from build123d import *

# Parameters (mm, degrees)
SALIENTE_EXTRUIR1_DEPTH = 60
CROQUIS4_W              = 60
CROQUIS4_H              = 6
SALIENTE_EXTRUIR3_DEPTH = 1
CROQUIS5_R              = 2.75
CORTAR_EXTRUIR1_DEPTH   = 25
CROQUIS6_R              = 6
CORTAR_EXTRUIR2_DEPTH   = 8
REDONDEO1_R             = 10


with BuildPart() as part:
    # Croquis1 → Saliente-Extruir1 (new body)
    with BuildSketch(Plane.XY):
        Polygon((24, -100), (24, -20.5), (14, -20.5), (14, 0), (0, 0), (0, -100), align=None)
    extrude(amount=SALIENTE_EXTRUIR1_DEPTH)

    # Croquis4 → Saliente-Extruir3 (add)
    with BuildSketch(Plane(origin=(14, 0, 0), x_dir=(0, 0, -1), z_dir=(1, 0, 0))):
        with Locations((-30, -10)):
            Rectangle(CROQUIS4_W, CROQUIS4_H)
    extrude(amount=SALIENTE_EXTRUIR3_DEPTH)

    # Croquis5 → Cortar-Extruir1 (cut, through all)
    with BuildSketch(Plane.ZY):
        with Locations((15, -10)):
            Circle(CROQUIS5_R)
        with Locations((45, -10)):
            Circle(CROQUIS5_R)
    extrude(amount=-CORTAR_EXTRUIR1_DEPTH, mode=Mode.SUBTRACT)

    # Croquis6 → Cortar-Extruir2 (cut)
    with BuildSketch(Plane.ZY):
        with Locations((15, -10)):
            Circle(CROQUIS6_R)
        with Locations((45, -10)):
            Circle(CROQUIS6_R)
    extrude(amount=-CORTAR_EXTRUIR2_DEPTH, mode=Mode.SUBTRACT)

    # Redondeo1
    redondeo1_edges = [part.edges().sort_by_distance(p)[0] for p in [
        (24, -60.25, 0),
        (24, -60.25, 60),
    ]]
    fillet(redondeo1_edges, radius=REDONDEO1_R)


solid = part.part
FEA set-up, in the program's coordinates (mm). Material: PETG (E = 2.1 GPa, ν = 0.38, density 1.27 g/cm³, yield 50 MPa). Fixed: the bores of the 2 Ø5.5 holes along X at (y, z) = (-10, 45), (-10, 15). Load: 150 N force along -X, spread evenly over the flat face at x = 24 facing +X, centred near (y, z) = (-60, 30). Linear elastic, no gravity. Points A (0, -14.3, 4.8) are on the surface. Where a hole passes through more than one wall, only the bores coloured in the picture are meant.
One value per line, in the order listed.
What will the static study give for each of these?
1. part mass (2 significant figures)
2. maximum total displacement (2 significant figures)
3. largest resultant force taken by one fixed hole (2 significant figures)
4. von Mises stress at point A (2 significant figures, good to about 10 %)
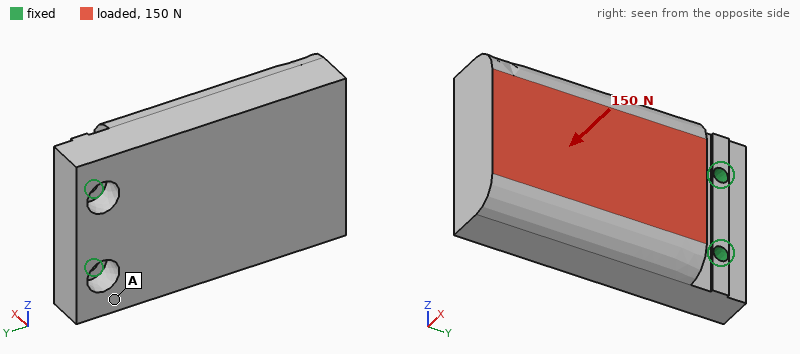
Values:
160 g
1.2 mm
80 N
3.7 MPa
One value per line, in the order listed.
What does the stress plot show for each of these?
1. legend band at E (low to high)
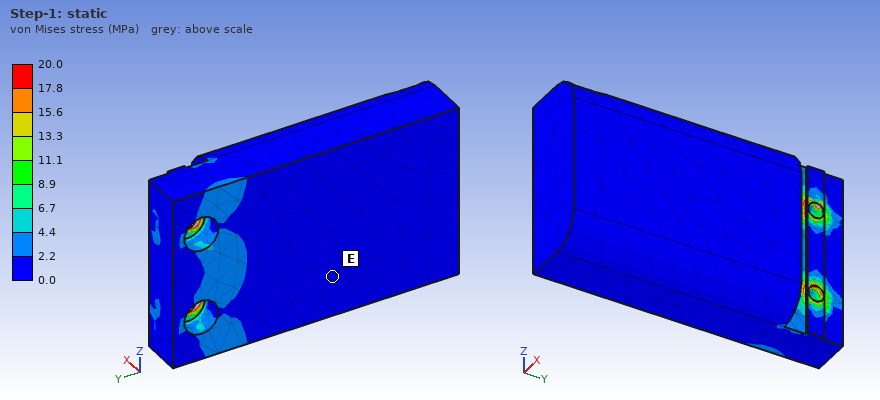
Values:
0.0 to 2.2 MPa
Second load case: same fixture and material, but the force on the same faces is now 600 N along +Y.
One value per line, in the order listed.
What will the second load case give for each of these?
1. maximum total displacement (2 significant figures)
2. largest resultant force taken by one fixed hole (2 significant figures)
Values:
1.4 mm
310 N
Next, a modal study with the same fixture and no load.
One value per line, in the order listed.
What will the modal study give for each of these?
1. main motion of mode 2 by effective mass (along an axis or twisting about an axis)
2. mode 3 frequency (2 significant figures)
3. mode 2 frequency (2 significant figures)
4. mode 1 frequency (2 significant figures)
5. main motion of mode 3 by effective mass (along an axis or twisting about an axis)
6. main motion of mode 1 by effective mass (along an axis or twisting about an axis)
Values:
along Z
1100 Hz
650 Hz
180 Hz
twisting about Y
along X
